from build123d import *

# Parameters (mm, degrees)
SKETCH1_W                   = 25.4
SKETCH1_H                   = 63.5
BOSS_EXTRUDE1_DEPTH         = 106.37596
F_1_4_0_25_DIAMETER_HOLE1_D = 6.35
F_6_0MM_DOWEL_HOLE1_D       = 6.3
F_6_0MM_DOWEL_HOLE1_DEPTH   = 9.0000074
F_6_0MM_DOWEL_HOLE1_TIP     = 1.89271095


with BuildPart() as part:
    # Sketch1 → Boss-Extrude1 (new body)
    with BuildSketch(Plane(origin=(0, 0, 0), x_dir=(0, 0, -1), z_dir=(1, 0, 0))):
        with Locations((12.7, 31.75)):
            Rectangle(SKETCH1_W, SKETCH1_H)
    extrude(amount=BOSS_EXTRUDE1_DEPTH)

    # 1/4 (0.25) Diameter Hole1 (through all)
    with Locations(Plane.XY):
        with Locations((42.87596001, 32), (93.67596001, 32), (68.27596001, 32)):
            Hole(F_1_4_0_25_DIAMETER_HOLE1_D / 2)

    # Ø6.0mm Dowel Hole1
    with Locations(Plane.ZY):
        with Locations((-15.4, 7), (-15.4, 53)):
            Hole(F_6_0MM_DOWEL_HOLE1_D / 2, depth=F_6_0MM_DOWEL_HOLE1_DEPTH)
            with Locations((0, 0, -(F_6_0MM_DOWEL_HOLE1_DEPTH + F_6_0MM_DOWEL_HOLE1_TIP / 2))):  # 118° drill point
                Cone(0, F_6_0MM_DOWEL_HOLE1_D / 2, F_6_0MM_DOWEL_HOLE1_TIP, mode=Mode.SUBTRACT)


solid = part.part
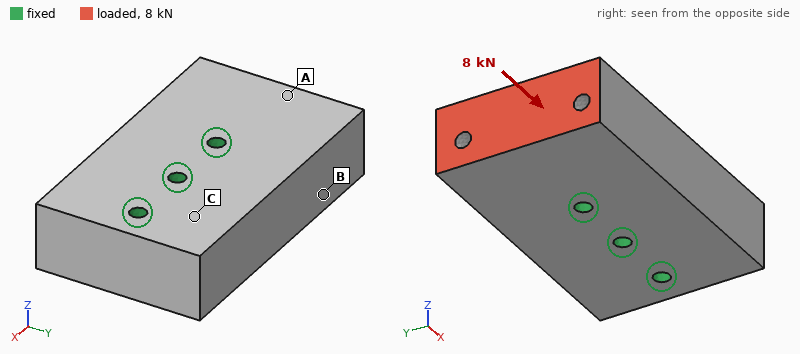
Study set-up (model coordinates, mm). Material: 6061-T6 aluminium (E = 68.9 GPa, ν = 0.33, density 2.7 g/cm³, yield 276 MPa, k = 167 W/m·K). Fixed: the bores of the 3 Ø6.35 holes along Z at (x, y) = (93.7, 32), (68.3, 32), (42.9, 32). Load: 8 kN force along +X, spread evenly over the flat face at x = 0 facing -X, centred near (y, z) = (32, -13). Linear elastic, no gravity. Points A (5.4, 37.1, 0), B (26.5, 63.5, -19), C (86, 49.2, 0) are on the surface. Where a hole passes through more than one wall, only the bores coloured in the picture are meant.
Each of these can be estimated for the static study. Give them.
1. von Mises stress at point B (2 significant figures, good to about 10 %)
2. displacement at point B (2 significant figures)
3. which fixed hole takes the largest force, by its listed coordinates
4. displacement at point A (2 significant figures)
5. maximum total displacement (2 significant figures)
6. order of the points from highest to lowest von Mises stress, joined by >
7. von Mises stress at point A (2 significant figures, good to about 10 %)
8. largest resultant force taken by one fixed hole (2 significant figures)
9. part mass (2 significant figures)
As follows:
3.5 MPa
2.9 µm
(42.9, 32)
3.9 µm
4.9 µm
A > B > C
5.6 MPa
5.2 kN
460 g
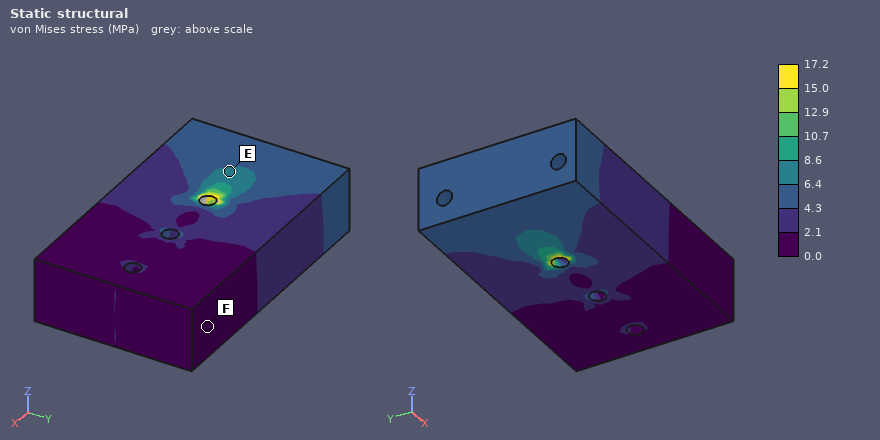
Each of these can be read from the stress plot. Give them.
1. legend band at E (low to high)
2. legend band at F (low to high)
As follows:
6.4 to 8.6 MPa
0.0 to 2.1 MPa
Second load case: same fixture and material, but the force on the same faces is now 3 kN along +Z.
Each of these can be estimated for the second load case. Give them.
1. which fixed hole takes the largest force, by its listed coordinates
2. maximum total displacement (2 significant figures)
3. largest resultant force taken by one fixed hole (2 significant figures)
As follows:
(42.9, 32)
26 µm
4.3 kN
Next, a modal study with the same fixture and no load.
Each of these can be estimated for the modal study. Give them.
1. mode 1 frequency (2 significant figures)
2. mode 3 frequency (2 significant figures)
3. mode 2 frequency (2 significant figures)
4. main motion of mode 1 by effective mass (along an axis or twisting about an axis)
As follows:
7100 Hz
8900 Hz
8600 Hz
along Z
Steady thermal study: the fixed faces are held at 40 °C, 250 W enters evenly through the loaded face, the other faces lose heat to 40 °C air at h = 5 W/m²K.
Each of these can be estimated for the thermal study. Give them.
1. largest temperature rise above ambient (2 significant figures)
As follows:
48 K
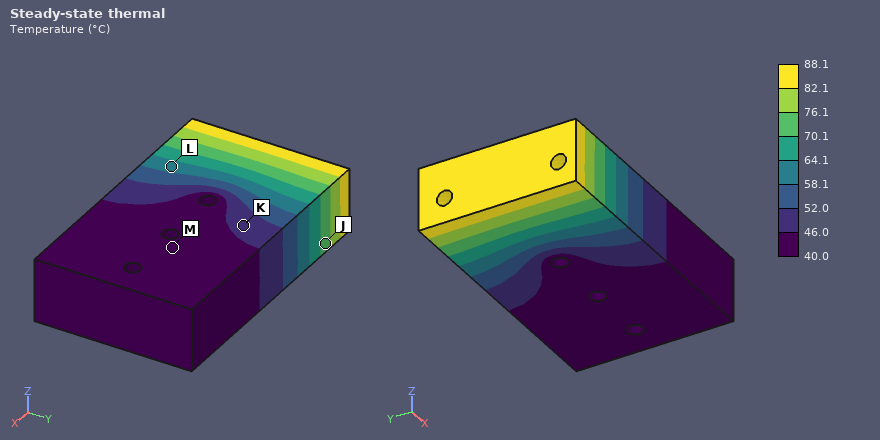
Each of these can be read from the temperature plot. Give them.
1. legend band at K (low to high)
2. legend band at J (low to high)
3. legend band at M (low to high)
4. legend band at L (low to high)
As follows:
46.0 to 52.0 °C
70.1 to 76.1 °C
40.0 to 46.0 °C
58.1 to 64.1 °C
